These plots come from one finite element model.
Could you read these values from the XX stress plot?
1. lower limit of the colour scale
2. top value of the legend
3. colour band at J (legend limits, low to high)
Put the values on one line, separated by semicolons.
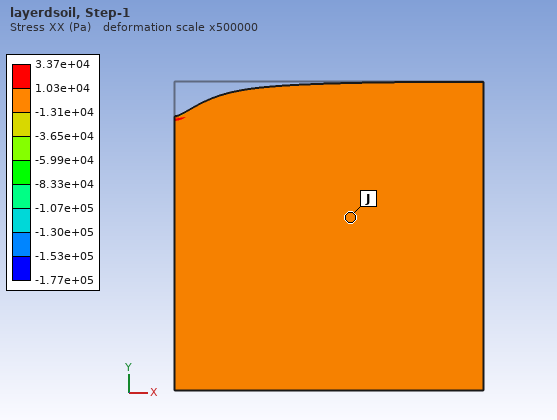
-1.77e+05 Pa; 3.37e+04 Pa; -1.31e+04 to 1.03e+04 Pa
